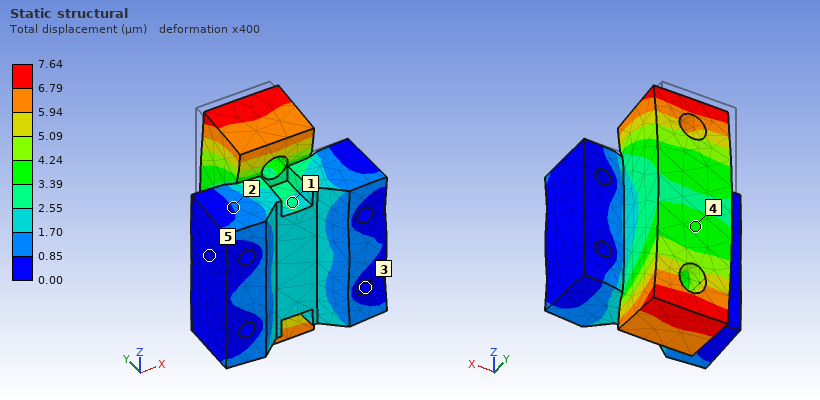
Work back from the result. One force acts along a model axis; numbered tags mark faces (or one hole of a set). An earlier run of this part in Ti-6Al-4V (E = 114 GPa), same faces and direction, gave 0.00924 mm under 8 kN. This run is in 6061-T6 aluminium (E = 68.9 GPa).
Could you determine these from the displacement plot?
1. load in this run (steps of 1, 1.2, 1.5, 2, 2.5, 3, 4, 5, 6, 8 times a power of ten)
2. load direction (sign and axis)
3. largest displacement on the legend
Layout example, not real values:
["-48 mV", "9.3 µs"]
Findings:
["4 kN", "-Y", "7.64 µm"]
